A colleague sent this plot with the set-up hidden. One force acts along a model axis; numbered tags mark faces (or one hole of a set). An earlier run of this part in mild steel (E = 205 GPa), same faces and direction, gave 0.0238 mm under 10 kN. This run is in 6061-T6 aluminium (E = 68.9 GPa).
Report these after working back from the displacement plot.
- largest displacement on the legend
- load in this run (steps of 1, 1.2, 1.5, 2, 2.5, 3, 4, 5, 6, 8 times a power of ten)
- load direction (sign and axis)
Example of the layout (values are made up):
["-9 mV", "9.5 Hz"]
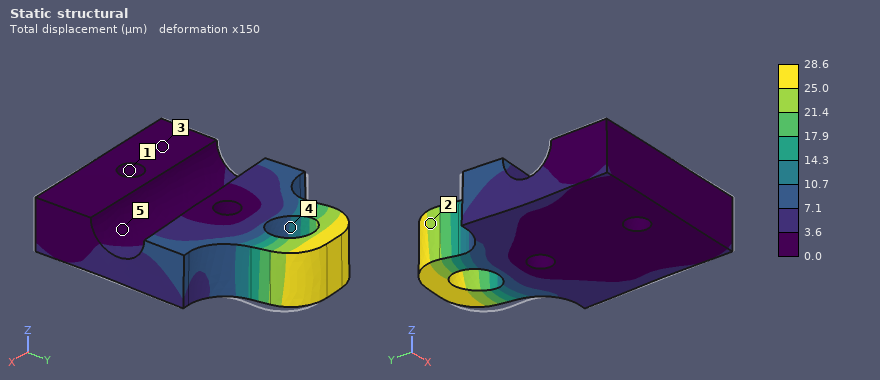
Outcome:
["28.6 µm", "4 kN", "-X"]
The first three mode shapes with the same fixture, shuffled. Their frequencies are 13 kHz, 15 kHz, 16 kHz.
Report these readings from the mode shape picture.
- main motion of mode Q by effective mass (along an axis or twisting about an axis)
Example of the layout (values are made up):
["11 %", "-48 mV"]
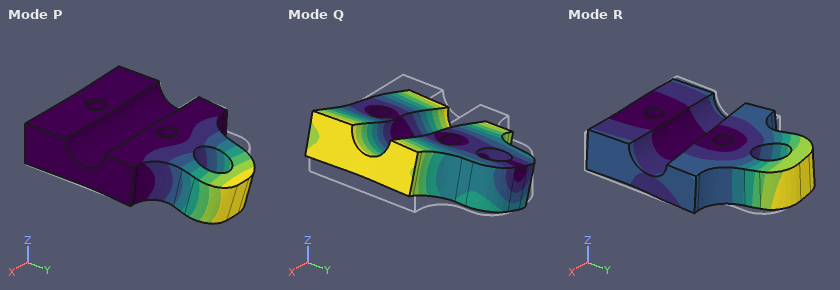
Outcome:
["twisting about Y"]
